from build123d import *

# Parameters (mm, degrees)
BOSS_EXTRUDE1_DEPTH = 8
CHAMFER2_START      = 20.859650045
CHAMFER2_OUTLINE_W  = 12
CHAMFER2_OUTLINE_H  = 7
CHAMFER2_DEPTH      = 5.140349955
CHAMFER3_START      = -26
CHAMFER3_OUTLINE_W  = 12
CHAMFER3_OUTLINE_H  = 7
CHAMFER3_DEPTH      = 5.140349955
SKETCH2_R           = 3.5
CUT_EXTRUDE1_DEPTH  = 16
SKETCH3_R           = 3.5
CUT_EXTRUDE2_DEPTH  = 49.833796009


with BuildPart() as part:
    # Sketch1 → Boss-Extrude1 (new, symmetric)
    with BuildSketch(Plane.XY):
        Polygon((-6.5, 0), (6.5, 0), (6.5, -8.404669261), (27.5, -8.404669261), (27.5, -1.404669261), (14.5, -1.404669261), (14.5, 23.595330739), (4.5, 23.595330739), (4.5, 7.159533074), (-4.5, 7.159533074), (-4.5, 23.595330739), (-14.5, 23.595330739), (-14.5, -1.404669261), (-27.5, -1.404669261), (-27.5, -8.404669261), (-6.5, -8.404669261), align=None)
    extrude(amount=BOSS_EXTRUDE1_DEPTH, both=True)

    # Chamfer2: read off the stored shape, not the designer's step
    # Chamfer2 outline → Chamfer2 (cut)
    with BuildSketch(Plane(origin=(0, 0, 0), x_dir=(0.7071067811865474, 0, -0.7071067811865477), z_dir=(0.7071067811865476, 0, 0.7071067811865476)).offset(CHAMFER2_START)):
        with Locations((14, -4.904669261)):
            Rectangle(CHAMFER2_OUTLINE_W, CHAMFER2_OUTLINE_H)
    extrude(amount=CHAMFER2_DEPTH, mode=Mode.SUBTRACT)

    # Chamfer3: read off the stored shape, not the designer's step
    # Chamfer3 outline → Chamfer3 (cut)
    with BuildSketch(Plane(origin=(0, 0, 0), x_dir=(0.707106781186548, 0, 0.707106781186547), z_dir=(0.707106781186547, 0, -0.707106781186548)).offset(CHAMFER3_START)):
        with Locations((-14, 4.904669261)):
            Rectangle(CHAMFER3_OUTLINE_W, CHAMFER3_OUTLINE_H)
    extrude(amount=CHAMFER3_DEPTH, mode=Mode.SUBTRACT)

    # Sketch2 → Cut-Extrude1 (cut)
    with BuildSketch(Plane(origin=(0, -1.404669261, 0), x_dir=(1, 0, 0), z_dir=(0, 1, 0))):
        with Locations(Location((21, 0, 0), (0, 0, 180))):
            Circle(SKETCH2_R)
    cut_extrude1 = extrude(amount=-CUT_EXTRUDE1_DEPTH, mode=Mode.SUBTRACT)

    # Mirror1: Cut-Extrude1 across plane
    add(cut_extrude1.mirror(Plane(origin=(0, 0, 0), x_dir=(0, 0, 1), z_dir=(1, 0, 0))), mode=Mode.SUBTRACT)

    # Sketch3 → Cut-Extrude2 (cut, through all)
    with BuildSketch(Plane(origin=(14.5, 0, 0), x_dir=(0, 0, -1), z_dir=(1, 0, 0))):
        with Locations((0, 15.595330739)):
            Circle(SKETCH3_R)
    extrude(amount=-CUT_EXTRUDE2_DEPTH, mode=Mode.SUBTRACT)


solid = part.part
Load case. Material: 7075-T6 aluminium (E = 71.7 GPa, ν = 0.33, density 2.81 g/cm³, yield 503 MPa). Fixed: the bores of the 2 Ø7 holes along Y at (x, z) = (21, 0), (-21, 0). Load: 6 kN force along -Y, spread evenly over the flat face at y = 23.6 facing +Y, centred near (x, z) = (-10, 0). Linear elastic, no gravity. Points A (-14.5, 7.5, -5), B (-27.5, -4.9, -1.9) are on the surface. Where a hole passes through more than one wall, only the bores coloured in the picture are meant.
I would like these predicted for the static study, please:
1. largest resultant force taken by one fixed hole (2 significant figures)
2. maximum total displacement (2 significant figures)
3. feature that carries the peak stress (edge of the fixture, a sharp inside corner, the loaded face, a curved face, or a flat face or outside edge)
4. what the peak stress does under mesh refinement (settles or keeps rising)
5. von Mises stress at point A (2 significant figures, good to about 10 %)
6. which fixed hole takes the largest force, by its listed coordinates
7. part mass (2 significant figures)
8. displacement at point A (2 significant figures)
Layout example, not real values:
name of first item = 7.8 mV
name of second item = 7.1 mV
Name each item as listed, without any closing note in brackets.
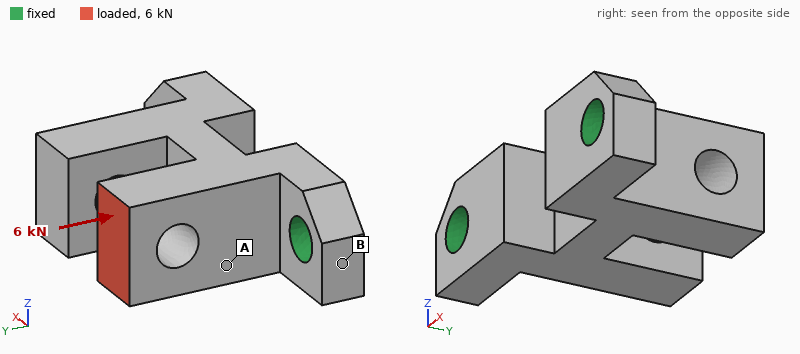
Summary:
largest resultant force taken by one fixed hole = 5.3 kN
maximum total displacement = 45 µm
feature that carries the peak stress = edge of the fixture
what the peak stress does under mesh refinement = keeps rising
von Mises stress at point A = 51 MPa
which fixed hole takes the largest force, by its listed coordinates = (-21, 0)
part mass = 34 g
displacement at point A = 27 µm
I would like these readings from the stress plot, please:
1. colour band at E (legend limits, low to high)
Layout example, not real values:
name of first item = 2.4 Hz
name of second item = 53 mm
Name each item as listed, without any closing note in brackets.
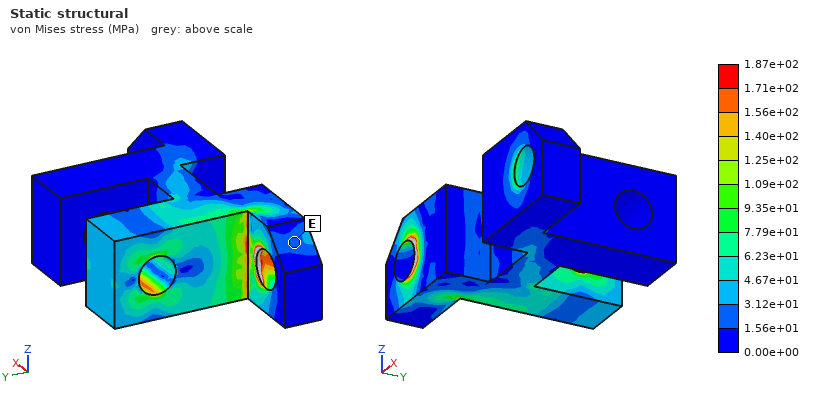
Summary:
colour band at E = 1.56e+01 to 3.12e+01 MPa
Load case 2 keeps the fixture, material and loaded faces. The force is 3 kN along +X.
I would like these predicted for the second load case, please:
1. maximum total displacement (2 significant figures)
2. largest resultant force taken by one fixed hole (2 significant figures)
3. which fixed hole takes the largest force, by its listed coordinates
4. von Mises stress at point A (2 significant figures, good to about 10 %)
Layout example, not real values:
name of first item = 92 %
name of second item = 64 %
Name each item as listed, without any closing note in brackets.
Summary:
maximum total displacement = 0.19 mm
largest resultant force taken by one fixed hole = 4.5 kN
which fixed hole takes the largest force, by its listed coordinates = (21, 0)
von Mises stress at point A = 170 MPa
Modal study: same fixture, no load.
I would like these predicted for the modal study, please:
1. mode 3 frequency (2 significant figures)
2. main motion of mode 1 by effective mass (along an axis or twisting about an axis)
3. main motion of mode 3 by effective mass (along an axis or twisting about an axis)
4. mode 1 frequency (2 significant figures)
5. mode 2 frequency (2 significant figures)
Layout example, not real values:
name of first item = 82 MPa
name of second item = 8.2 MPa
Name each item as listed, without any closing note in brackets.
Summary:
mode 3 frequency = 13 kHz
main motion of mode 1 by effective mass = along Z
main motion of mode 3 by effective mass = along X
mode 1 frequency = 6200 Hz
mode 2 frequency = 11 kHz
